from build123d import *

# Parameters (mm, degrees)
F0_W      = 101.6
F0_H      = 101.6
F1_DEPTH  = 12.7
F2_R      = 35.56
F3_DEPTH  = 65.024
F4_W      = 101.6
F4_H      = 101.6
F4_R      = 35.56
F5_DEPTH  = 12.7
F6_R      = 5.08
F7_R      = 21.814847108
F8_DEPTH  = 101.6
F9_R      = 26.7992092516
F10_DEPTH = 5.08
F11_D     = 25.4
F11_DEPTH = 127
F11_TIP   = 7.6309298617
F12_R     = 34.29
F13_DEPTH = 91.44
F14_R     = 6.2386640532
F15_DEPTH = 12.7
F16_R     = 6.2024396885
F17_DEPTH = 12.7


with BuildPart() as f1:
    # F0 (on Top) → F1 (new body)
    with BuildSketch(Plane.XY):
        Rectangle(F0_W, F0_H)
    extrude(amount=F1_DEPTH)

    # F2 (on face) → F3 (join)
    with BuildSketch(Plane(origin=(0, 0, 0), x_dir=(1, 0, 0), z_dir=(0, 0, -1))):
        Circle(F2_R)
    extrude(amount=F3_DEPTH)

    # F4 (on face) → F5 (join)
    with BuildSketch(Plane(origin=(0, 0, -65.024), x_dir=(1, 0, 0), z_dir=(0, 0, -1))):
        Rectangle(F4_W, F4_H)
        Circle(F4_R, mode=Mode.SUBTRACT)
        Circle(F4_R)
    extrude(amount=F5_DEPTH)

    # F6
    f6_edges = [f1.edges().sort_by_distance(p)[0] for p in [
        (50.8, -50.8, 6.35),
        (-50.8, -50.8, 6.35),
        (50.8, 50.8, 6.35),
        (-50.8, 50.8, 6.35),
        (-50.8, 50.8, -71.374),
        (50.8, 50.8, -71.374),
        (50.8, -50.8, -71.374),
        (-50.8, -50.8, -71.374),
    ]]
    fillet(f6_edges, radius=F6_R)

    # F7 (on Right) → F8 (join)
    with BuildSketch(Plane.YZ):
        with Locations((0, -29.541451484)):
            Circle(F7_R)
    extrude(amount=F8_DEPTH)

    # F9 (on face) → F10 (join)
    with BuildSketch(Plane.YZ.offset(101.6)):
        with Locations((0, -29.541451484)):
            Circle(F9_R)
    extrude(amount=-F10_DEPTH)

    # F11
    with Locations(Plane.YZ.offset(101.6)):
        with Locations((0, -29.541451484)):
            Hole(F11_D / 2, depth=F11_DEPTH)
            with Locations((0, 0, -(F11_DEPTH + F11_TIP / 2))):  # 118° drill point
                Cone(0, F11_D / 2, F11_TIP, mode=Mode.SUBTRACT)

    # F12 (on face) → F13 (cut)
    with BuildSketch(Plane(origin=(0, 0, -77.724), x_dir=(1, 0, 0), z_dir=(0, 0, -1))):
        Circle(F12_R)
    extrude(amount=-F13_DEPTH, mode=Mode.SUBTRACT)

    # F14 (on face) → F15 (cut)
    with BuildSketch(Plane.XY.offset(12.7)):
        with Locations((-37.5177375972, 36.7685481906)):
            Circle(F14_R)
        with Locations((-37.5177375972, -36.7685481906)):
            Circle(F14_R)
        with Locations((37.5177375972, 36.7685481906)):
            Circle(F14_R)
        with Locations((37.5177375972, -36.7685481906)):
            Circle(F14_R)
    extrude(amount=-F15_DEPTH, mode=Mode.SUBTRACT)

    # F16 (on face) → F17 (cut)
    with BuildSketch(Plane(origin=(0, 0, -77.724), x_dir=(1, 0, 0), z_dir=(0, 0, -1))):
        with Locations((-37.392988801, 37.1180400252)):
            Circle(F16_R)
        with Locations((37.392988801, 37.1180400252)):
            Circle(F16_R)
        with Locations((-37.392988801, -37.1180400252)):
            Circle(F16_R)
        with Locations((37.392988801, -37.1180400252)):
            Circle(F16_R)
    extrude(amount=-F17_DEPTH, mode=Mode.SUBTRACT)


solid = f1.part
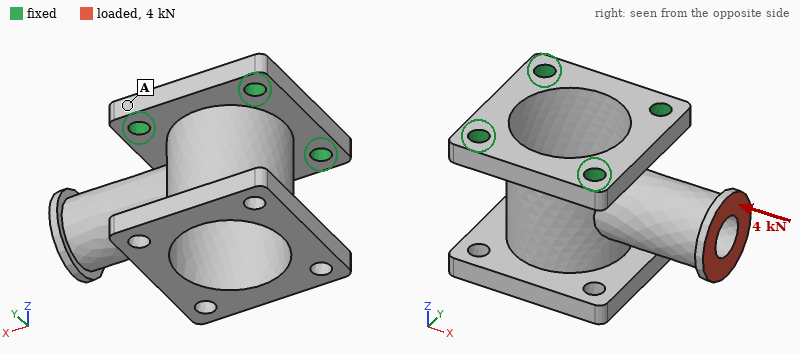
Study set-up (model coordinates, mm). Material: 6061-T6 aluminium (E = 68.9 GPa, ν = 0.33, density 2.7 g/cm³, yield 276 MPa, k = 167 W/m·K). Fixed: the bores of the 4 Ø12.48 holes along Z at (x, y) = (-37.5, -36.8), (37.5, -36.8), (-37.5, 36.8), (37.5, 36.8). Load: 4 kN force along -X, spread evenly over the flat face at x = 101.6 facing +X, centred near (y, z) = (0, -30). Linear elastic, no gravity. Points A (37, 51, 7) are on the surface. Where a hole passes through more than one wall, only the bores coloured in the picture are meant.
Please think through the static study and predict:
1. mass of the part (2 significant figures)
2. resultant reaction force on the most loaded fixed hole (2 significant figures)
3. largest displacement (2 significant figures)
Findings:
660 g
2.0 kN
0.18 mm
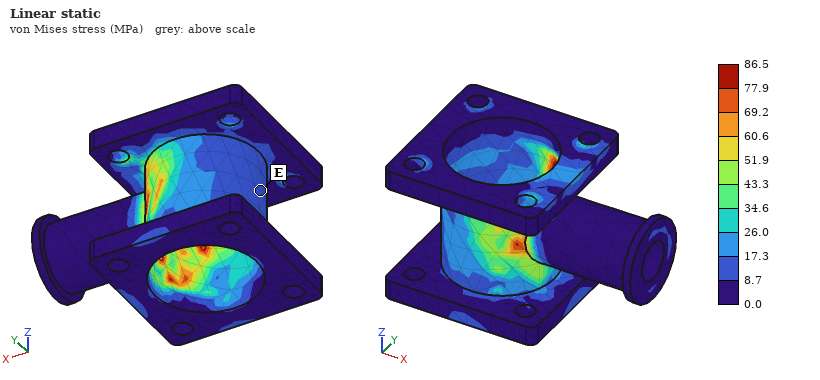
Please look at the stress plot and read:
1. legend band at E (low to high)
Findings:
8.7 to 17.3 MPa
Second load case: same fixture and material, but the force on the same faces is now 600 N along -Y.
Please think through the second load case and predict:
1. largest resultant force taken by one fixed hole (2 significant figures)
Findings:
670 N
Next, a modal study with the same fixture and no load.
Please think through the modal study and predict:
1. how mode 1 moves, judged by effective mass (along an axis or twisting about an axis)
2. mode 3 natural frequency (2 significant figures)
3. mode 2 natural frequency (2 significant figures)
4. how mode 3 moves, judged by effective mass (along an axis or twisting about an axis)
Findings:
along Y
1600 Hz
1100 Hz
along Y
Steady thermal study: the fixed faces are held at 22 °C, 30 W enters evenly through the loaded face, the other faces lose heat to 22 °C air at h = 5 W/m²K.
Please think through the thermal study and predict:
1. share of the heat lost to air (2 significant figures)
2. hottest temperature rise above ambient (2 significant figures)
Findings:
17 %
34 K
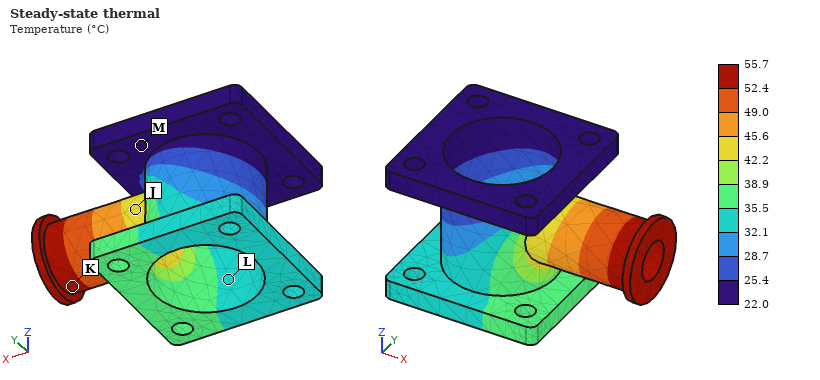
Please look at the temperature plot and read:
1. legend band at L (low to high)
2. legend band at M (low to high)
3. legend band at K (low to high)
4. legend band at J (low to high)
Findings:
32.1 to 35.5 °C
22.0 to 25.4 °C
52.4 to 55.7 °C
42.2 to 45.6 °C
